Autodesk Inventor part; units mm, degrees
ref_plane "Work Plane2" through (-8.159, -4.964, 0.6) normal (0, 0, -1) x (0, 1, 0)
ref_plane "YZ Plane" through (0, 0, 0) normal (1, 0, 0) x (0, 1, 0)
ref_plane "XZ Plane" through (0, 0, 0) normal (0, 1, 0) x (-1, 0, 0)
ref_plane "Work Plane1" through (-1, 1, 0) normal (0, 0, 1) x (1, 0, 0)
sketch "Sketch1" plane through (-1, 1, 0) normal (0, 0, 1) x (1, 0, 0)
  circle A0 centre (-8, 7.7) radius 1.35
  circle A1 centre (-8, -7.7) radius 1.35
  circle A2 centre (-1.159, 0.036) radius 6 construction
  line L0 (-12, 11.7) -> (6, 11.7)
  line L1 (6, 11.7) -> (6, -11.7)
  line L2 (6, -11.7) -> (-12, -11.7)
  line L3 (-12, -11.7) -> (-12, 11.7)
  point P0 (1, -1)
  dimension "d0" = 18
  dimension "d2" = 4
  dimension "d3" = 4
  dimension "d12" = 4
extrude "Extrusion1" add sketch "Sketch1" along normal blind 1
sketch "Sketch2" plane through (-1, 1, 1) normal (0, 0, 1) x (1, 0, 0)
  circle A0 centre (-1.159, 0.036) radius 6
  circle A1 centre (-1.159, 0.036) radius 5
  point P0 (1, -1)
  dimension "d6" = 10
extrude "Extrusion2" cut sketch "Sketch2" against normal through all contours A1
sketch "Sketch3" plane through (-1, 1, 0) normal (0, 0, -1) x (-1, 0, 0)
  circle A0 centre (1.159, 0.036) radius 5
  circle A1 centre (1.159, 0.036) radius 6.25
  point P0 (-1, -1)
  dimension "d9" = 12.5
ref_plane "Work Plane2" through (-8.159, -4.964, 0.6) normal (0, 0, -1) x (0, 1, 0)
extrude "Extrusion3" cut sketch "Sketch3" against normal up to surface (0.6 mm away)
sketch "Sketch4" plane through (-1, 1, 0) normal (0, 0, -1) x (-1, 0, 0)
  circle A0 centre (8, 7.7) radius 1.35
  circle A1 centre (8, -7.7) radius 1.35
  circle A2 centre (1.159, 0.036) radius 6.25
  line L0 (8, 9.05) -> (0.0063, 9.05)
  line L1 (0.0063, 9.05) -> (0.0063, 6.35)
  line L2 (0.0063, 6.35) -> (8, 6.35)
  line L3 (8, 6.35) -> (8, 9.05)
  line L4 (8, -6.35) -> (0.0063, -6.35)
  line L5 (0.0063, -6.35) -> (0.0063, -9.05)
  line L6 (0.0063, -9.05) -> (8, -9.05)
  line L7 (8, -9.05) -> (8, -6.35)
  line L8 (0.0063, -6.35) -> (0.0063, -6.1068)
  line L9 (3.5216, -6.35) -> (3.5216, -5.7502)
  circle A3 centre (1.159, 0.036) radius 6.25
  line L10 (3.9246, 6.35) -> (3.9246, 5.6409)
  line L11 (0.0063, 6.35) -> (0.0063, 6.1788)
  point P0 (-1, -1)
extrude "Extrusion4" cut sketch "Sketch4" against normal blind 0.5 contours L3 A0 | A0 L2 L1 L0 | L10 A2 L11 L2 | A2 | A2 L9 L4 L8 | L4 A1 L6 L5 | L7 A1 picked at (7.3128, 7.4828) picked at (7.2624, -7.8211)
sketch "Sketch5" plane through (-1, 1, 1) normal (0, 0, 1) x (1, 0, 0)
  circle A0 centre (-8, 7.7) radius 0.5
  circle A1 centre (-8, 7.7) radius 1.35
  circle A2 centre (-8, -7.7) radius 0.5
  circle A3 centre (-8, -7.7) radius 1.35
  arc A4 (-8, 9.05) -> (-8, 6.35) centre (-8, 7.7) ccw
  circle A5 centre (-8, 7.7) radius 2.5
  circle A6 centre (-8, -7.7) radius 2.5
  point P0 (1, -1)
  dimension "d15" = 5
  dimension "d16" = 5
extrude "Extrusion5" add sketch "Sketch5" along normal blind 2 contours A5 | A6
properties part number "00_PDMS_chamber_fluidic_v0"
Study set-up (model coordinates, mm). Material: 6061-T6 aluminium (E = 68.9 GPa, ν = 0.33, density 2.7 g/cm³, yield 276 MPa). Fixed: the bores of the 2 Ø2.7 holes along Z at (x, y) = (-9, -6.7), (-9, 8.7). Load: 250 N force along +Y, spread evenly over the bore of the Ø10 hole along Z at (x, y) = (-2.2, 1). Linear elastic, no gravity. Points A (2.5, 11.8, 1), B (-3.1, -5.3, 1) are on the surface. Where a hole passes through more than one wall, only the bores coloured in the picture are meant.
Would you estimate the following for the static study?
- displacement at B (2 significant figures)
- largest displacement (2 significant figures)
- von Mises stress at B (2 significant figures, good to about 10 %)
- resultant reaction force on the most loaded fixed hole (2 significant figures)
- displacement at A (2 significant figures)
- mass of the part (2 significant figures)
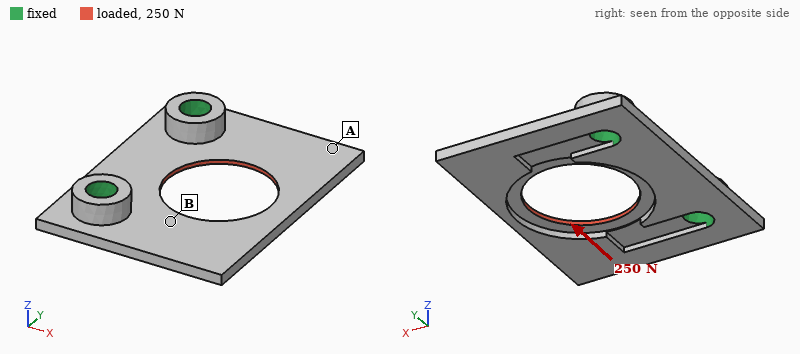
8.1 µm
28 µm
47 MPa
140 N
22 µm
0.92 g
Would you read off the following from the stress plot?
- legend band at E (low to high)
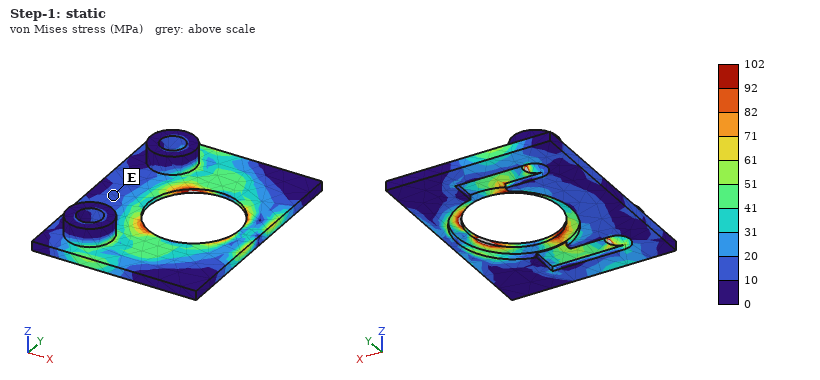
10 to 20 MPa
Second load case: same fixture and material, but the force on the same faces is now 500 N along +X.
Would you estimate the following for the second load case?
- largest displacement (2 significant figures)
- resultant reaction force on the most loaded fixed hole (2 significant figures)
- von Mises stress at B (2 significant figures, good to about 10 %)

59 µm
260 N
77 MPa
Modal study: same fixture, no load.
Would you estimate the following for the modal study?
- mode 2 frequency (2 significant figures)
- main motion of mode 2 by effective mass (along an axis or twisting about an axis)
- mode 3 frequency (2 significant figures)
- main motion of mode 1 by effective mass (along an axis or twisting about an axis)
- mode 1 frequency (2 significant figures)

5400 Hz
twisting about X
12 kHz
along Z
3400 Hz
